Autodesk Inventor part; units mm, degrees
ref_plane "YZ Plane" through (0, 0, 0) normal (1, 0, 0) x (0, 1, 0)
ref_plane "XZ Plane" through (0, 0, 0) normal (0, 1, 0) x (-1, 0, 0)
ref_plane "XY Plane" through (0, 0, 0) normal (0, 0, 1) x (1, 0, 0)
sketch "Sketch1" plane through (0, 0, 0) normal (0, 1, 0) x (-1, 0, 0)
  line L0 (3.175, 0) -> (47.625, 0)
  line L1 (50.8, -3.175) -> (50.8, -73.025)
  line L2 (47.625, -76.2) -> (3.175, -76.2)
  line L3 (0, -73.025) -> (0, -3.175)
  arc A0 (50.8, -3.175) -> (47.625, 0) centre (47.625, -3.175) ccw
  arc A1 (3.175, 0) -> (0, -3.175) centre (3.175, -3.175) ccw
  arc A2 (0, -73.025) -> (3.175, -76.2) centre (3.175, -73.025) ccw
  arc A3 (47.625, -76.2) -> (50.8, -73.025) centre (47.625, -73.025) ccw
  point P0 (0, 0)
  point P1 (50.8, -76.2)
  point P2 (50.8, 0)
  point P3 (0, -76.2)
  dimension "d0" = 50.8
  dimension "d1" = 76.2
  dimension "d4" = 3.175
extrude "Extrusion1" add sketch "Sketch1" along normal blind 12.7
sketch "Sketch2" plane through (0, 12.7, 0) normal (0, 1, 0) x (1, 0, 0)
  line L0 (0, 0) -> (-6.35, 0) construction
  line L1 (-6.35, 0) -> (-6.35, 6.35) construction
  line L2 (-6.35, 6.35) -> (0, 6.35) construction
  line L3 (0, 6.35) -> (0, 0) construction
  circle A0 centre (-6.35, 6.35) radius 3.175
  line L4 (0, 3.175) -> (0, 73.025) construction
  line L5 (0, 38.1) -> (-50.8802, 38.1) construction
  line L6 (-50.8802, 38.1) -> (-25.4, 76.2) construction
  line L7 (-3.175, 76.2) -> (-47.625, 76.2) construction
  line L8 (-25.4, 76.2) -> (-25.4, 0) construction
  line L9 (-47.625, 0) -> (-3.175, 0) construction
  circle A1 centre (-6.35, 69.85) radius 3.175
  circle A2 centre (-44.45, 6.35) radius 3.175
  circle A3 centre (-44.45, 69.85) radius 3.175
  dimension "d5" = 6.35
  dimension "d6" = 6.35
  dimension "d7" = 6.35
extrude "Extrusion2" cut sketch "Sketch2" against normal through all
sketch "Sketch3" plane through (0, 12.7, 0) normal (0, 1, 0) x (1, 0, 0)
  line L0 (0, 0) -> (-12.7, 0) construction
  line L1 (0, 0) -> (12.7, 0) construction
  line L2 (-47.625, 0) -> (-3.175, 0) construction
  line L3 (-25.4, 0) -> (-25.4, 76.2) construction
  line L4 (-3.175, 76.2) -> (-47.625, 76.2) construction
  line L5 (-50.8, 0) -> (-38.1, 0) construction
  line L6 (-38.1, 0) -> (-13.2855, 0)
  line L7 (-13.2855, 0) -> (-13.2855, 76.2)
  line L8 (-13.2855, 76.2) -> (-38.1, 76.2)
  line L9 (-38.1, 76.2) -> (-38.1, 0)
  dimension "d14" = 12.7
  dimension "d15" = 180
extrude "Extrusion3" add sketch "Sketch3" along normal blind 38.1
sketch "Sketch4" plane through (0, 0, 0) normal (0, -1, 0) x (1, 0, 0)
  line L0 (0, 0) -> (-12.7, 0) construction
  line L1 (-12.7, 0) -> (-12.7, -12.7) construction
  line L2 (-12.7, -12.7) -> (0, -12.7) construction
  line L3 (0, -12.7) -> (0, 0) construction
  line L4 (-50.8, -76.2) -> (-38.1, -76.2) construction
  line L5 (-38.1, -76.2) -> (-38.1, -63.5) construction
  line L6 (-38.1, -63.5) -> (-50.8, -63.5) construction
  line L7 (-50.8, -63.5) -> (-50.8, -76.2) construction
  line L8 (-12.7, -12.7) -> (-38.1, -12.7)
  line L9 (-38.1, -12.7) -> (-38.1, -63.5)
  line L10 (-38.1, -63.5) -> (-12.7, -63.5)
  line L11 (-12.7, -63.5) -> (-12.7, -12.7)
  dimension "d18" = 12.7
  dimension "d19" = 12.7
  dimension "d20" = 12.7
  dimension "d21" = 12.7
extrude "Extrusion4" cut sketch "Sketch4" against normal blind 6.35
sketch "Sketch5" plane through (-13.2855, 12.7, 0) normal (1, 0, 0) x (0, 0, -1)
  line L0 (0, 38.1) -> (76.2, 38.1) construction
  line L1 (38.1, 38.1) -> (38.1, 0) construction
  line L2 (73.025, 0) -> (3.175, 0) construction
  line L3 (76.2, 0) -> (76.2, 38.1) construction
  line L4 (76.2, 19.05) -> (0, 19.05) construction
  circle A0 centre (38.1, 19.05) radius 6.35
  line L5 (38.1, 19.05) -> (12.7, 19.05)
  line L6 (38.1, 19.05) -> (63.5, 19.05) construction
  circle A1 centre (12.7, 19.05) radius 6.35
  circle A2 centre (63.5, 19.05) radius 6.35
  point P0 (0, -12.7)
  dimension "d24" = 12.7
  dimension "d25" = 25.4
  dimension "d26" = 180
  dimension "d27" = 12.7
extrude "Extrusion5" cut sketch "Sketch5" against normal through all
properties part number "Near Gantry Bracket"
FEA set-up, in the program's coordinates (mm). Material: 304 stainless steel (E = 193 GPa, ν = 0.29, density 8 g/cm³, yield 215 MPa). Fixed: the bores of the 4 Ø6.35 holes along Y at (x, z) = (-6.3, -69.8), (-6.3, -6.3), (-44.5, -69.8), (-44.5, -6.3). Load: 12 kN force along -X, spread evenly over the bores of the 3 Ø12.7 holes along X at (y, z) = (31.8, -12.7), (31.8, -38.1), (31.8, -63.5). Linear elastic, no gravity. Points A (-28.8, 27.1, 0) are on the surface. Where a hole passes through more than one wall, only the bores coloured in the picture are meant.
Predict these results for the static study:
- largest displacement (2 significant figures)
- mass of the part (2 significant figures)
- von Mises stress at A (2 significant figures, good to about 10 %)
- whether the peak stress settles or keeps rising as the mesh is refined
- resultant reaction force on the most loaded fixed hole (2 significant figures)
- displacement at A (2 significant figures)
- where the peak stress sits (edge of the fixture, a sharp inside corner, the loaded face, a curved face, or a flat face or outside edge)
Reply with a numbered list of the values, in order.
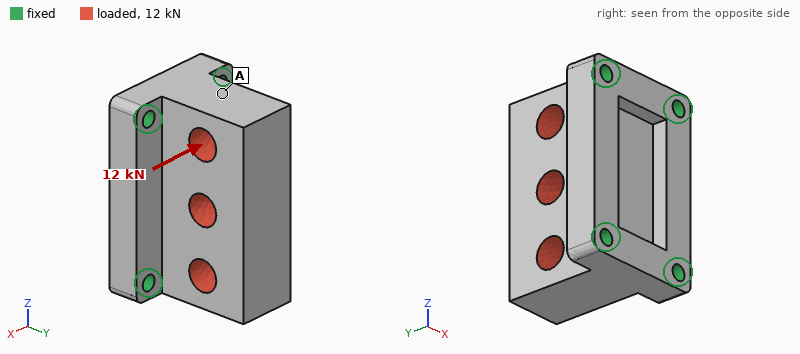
1. 21 µm
2. 810 g
3. 18 MPa
4. keeps rising
5. 5.6 kN
6. 7.2 µm
7. edge of the fixture
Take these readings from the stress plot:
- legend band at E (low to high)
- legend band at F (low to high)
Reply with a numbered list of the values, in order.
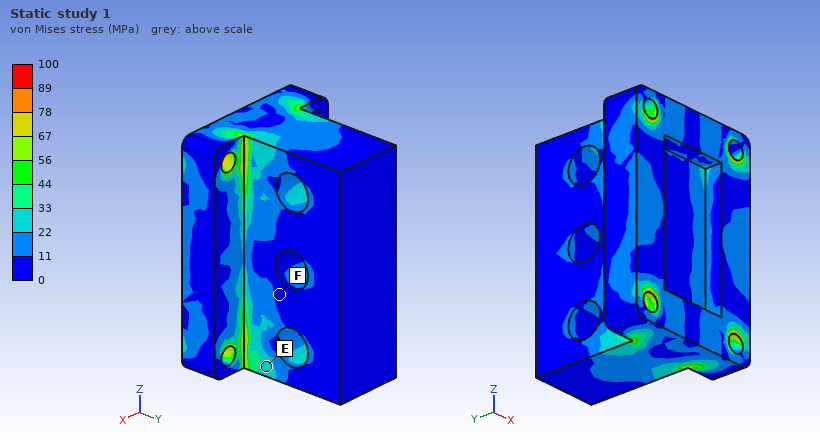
1. 22 to 33 MPa
2. 0 to 11 MPa
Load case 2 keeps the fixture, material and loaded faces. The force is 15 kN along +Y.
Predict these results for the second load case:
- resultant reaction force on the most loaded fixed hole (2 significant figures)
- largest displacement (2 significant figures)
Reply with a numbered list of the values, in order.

1. 4.2 kN
2. 5.4 µm
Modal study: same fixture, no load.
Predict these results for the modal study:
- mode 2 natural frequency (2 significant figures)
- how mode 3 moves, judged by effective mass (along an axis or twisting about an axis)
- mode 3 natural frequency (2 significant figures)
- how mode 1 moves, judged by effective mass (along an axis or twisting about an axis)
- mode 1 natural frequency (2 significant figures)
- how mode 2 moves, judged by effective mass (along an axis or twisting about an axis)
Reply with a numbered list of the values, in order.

1. 9300 Hz
2. twisting about Y
3. 11 kHz
4. along X
5. 6100 Hz
6. along Z
